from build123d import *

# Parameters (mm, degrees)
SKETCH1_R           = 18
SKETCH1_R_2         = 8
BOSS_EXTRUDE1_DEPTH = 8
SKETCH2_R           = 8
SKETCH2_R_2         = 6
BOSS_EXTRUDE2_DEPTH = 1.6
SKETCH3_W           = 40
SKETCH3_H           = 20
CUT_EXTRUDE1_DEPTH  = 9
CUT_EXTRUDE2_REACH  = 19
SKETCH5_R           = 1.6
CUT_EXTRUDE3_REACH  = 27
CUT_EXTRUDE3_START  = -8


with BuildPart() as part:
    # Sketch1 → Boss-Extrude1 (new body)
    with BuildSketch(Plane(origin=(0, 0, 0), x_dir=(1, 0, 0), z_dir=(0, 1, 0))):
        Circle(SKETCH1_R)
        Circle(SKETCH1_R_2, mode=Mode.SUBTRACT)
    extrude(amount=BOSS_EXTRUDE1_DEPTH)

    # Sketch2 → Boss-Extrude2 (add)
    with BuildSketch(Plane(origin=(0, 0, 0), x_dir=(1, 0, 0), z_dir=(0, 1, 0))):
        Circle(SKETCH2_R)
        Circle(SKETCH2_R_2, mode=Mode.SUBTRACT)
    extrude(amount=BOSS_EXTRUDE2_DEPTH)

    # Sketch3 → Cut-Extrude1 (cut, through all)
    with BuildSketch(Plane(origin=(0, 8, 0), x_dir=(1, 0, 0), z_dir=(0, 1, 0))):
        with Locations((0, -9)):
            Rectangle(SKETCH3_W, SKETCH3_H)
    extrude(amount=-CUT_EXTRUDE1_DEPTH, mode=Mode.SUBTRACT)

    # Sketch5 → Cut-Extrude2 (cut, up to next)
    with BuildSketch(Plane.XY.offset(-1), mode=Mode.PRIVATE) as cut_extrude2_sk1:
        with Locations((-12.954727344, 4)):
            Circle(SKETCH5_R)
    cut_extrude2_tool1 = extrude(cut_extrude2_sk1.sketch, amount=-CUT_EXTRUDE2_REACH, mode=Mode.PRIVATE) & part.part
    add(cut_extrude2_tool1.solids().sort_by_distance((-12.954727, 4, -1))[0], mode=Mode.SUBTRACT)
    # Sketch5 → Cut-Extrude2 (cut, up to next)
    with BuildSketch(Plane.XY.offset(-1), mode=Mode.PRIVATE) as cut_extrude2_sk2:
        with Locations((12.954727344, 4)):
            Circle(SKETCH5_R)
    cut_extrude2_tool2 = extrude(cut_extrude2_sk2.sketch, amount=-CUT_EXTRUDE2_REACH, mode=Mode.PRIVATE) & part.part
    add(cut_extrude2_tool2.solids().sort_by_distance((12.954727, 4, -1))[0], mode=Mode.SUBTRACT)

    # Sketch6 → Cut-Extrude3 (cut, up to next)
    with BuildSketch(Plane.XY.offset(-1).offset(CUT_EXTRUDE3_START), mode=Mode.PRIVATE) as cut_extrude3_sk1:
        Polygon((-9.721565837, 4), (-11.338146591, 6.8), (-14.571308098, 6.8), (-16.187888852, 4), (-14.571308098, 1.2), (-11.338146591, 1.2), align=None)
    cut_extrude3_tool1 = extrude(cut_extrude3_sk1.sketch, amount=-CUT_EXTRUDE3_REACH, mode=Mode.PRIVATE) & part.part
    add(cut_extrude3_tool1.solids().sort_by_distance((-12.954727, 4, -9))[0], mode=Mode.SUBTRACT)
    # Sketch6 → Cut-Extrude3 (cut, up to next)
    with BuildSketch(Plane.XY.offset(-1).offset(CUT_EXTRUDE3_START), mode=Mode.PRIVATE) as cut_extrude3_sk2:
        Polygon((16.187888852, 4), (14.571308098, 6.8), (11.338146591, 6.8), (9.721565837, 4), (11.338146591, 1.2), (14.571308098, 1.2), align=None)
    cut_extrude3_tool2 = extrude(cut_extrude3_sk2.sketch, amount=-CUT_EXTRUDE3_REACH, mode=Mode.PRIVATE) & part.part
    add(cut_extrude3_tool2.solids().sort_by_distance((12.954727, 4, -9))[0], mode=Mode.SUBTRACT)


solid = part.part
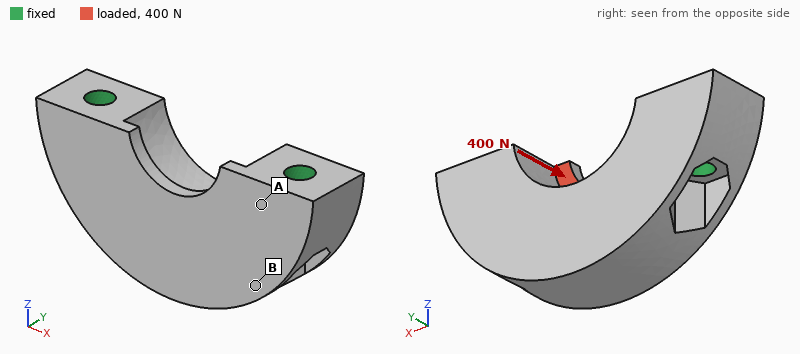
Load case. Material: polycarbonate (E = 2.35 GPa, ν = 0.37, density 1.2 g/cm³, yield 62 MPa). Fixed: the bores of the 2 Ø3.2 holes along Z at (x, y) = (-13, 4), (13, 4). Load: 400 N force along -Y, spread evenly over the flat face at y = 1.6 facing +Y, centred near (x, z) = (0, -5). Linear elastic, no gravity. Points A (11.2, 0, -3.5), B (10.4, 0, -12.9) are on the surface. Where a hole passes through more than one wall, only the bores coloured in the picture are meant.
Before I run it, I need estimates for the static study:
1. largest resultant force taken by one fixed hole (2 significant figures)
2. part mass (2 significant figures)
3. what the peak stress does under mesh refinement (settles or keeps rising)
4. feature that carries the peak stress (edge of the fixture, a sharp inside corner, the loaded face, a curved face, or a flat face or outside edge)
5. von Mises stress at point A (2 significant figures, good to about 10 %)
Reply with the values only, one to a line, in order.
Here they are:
200 N
3.4 g
keeps rising
a sharp inside corner
9.6 MPa
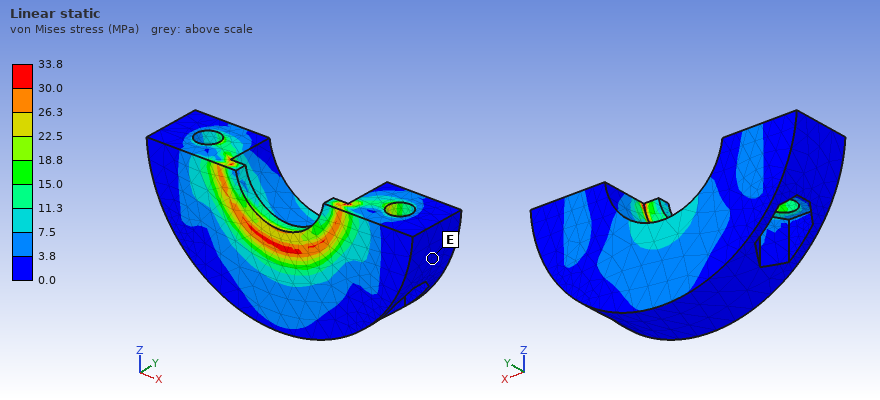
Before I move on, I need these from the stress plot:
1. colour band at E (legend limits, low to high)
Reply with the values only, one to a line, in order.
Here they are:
0.0 to 3.8 MPa
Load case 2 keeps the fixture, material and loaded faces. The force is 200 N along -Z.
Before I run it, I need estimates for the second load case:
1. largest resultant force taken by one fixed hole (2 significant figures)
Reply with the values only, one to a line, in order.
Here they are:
110 N
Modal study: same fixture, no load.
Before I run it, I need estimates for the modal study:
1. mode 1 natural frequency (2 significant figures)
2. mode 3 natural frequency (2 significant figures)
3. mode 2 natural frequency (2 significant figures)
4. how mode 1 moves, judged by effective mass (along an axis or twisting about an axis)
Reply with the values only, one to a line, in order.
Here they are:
5900 Hz
14 kHz
13 kHz
along Y
